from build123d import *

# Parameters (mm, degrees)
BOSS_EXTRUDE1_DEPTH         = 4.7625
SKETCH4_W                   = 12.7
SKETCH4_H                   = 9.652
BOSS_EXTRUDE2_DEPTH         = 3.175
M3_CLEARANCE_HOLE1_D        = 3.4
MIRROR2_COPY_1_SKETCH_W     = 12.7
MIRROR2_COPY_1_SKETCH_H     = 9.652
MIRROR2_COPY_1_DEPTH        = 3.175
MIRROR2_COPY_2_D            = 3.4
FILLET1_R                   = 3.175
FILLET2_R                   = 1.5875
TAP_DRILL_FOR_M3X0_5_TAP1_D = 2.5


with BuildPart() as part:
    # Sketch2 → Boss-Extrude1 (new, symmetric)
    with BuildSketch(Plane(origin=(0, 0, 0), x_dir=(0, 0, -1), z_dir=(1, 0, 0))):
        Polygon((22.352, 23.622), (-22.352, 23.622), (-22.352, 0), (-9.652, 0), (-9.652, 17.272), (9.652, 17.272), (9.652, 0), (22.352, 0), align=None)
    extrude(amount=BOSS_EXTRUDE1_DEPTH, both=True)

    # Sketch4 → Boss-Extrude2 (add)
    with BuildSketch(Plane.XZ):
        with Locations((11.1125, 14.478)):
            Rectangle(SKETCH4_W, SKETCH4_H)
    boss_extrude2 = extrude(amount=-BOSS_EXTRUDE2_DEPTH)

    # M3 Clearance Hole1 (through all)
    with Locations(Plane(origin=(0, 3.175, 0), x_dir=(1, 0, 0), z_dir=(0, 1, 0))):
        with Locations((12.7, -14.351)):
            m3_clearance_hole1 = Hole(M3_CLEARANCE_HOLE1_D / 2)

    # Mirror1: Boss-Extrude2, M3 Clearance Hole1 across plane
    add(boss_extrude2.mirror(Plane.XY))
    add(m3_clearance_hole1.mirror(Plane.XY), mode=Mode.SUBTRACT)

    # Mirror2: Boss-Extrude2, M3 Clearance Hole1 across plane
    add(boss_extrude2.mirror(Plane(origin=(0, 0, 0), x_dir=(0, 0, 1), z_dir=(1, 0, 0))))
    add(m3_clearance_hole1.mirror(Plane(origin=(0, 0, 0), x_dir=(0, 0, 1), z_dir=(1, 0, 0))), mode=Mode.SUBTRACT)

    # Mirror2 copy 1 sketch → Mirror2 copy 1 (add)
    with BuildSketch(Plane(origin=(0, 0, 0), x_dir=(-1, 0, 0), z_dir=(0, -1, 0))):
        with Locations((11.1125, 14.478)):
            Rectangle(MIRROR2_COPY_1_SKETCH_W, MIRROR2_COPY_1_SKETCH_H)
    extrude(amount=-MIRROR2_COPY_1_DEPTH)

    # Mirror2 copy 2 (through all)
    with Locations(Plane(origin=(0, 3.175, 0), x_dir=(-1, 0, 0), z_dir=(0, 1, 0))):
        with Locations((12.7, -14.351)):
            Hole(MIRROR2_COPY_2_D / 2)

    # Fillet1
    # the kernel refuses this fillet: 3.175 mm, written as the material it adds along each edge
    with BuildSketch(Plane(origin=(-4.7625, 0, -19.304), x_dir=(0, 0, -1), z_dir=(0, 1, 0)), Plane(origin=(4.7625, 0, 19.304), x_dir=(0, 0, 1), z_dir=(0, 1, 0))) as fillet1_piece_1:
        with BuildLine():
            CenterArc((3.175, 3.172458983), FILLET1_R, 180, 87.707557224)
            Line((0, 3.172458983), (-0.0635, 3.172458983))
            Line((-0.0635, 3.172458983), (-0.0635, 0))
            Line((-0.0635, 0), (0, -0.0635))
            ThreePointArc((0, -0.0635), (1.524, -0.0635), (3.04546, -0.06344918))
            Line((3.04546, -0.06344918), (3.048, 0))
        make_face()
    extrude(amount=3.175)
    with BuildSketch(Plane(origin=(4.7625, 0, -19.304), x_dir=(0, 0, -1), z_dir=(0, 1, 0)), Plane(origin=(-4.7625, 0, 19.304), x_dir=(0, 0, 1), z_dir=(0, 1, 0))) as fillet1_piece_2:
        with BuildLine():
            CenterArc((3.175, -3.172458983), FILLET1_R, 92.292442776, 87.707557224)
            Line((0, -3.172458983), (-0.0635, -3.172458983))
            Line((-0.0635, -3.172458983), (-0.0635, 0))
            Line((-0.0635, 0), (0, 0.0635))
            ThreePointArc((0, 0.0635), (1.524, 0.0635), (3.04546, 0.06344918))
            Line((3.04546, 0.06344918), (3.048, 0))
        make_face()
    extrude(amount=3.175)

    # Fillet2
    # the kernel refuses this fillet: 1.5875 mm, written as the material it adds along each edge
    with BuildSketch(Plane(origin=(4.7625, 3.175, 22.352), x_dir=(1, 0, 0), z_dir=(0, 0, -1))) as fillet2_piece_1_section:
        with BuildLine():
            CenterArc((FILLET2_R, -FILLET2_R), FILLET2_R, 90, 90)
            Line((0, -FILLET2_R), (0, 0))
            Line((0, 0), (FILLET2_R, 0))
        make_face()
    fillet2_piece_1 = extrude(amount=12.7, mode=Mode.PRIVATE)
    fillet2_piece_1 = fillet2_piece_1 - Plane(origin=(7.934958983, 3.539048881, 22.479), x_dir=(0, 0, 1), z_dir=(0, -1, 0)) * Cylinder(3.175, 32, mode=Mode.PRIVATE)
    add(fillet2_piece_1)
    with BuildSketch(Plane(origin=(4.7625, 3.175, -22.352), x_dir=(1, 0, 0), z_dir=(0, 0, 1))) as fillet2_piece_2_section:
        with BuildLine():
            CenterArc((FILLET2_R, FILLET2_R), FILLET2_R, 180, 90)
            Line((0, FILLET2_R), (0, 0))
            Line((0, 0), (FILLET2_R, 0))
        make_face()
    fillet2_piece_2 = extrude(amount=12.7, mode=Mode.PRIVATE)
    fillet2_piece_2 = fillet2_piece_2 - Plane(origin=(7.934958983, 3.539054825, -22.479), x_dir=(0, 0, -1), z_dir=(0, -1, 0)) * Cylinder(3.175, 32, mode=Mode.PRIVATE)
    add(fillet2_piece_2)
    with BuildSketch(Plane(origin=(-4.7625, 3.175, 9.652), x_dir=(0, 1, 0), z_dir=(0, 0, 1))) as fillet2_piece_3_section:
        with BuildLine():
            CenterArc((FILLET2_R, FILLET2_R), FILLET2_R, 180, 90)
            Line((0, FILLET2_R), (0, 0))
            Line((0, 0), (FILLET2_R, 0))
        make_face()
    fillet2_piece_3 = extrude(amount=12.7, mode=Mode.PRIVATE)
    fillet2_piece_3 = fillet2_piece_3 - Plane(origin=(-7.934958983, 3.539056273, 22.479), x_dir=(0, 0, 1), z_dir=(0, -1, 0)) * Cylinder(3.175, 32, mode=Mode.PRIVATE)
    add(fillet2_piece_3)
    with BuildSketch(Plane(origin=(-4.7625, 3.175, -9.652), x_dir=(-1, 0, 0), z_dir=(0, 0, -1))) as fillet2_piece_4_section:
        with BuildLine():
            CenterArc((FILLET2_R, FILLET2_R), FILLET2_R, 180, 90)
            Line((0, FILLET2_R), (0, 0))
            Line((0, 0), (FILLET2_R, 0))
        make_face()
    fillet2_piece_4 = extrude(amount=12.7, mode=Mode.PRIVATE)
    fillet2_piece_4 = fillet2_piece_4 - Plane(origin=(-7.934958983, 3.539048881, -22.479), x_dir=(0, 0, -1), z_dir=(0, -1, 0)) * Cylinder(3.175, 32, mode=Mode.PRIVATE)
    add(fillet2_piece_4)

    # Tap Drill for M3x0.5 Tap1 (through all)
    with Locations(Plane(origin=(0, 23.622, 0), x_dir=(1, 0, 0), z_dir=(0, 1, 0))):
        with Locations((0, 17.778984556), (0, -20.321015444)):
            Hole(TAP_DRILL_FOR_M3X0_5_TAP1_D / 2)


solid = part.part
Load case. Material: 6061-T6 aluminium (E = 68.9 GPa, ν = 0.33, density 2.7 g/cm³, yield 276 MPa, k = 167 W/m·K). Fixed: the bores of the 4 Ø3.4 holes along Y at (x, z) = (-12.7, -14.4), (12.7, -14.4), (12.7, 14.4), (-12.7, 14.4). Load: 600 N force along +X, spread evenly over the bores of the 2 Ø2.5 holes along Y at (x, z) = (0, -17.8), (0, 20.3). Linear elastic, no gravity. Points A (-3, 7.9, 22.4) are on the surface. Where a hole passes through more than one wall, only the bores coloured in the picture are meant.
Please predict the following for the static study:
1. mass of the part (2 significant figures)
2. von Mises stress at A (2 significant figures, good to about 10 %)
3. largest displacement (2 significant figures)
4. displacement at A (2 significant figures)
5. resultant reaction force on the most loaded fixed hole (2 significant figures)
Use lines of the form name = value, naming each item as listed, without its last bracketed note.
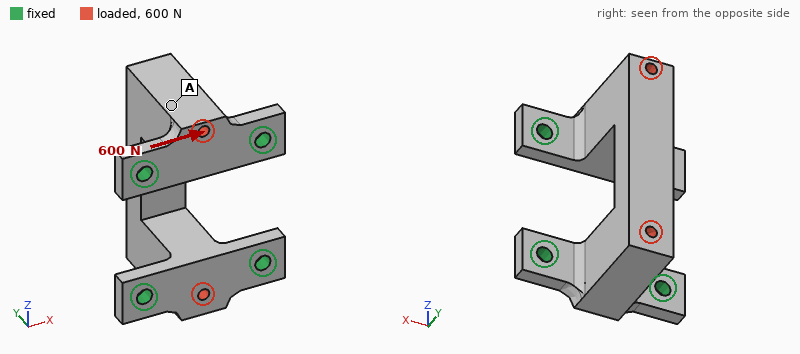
mass of the part = 22 g
von Mises stress at A = 6.1 MPa
largest displacement = 23 µm
displacement at A = 6.8 µm
resultant reaction force on the most loaded fixed hole = 240 N
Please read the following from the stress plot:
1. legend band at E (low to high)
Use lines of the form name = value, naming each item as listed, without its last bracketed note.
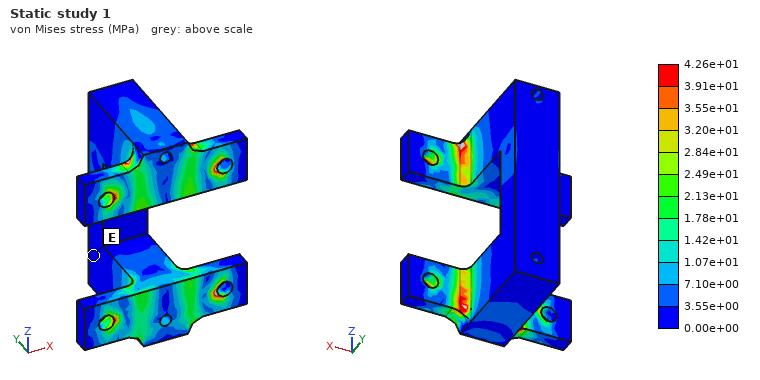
legend band at E = 0.00e+00 to 3.55e+00 MPa
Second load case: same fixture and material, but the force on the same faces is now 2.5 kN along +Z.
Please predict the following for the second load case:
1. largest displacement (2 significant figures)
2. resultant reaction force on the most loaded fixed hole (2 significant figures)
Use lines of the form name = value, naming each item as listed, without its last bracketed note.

largest displacement = 0.11 mm
resultant reaction force on the most loaded fixed hole = 710 N
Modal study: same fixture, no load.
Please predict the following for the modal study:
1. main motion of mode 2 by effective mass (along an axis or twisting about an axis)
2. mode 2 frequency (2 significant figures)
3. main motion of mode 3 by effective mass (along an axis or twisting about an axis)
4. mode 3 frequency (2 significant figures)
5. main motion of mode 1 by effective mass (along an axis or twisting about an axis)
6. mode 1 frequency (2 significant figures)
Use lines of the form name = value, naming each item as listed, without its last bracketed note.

main motion of mode 2 by effective mass = along X
mode 2 frequency = 6900 Hz
main motion of mode 3 by effective mass = twisting about Y
mode 3 frequency = 12 kHz
main motion of mode 1 by effective mass = along Z
mode 1 frequency = 6100 Hz
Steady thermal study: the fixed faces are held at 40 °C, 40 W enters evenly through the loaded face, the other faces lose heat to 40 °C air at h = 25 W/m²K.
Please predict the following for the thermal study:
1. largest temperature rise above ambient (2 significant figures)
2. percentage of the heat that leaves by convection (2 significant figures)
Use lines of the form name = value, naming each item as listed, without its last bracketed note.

largest temperature rise above ambient = 27 K
percentage of the heat that leaves by convection = 4.3 %
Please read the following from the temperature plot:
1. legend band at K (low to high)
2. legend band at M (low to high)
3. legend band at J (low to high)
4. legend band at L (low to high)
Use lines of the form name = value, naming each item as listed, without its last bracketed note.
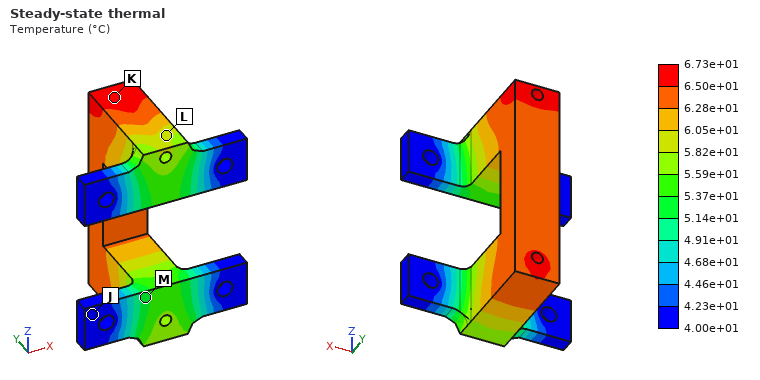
legend band at K = 6.50e+01 to 6.73e+01 °C
legend band at M = 5.14e+01 to 5.37e+01 °C
legend band at J = 4.00e+01 to 4.23e+01 °C
legend band at L = 5.82e+01 to 6.05e+01 °C
